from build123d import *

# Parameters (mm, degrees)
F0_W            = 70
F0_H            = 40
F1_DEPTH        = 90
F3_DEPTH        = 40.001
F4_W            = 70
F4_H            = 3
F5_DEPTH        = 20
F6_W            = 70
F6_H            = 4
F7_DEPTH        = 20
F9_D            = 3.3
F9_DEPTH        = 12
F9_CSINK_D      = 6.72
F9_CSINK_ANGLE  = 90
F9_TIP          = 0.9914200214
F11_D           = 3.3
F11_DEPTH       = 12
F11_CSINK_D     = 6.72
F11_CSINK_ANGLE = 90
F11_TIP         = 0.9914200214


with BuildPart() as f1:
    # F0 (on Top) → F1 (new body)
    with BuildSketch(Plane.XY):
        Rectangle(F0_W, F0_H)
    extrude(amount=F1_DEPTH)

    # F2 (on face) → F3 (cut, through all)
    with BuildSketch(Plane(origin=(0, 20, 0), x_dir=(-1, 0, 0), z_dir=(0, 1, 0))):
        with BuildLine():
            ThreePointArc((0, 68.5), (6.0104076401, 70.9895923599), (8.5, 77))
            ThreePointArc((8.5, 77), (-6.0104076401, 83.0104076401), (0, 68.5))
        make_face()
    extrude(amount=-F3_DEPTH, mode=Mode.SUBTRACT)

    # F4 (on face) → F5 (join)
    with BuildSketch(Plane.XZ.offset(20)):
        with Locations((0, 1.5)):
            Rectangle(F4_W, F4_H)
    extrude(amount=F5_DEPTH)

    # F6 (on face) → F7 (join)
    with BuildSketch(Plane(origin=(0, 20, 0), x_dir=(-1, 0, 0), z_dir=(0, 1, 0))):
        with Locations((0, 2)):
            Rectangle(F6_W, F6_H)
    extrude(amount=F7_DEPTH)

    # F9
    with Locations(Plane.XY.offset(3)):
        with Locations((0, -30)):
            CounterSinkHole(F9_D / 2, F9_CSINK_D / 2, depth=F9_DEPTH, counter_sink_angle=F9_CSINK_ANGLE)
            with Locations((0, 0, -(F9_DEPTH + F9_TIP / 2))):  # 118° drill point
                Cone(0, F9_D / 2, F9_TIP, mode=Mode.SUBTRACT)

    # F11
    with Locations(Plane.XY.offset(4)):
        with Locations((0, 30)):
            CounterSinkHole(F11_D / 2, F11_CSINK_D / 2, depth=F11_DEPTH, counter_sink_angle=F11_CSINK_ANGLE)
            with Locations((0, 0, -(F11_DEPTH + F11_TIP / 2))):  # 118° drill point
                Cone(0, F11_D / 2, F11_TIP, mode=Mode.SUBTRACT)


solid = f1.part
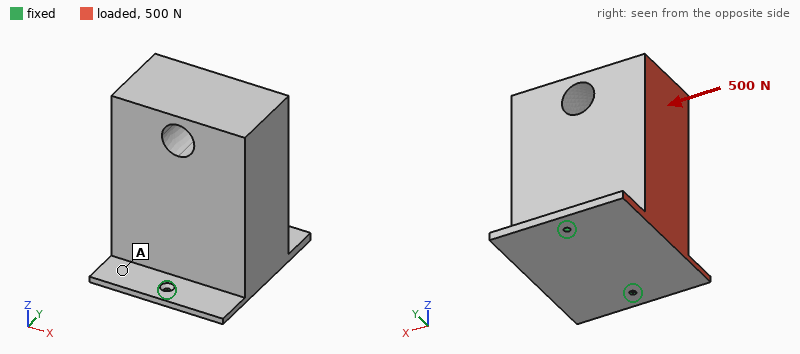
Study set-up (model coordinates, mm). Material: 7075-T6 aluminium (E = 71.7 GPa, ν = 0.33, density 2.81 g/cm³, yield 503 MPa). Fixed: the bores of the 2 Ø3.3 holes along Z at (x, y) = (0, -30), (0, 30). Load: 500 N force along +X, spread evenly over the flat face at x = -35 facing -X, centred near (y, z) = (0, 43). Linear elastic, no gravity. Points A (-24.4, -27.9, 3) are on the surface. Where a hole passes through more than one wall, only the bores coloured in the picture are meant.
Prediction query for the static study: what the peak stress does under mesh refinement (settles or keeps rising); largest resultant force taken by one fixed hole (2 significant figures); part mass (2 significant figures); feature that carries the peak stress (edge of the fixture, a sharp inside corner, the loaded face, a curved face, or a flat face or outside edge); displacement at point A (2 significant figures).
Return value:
keeps rising
260 N
710 g
edge of the fixture
0.35 mm
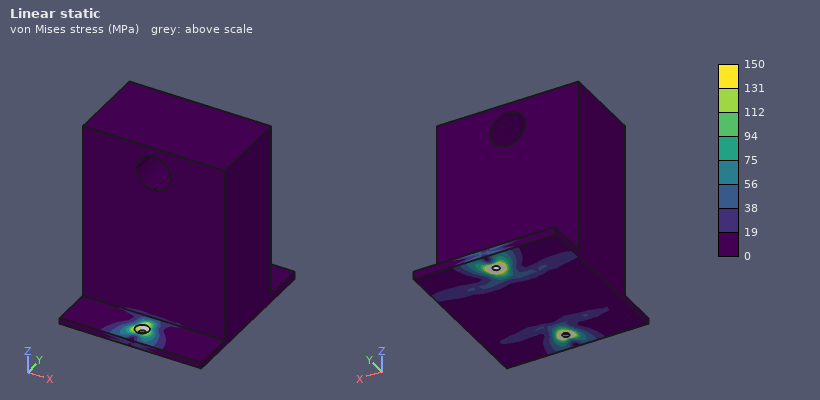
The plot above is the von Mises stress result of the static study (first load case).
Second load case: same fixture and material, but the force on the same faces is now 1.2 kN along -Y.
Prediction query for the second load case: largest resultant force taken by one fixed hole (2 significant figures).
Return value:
1.3 kN
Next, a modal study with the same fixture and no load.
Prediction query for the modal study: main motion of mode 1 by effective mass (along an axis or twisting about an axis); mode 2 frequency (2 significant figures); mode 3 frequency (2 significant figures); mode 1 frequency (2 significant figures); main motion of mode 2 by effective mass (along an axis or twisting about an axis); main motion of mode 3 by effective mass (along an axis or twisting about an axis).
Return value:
along X
660 Hz
1400 Hz
130 Hz
along Y
along Z
